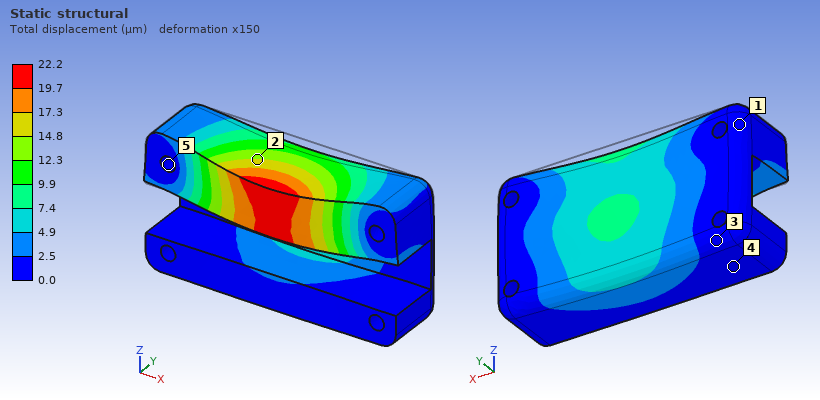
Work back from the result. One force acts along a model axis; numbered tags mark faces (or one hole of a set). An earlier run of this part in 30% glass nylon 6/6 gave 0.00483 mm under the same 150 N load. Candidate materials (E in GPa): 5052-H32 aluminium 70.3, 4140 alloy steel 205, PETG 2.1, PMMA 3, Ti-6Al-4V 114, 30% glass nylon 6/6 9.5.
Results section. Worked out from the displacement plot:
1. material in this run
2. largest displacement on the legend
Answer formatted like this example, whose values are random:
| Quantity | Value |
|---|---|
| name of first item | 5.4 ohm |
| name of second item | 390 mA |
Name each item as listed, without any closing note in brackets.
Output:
| Quantity | Value |
|---|---|
| material in this run | PETG |
| largest displacement on the legend | 22.2 µm |
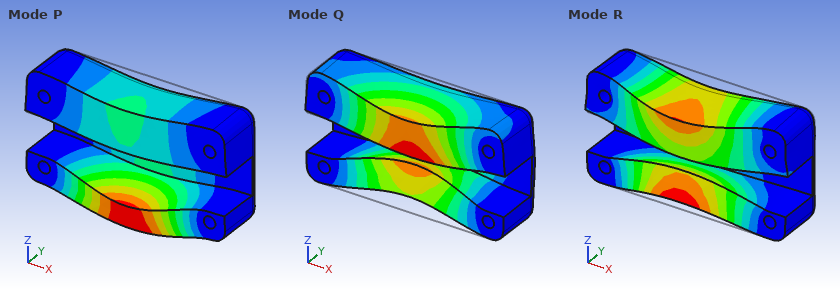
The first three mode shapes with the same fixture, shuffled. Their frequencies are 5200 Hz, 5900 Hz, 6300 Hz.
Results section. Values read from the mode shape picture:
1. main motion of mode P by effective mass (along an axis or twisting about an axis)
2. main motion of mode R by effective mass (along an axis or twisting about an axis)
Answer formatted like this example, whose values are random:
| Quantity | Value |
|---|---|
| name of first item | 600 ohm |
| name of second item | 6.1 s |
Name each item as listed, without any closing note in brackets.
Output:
| Quantity | Value |
|---|---|
| main motion of mode P by effective mass | along Z |
| main motion of mode R by effective mass | along Y |
